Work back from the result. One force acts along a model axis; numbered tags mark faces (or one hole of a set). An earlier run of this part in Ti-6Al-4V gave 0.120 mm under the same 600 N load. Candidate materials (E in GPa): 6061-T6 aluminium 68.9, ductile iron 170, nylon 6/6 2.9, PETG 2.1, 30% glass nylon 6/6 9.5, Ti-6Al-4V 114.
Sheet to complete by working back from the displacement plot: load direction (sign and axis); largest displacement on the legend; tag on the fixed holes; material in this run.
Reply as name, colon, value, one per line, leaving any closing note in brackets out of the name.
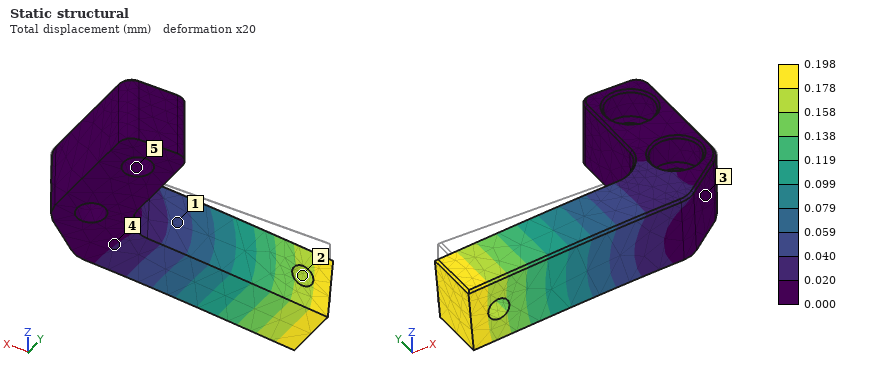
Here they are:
load direction: -Z
largest displacement on the legend: 0.198 mm
tag on the fixed holes: 5
material in this run: 6061-T6 aluminium
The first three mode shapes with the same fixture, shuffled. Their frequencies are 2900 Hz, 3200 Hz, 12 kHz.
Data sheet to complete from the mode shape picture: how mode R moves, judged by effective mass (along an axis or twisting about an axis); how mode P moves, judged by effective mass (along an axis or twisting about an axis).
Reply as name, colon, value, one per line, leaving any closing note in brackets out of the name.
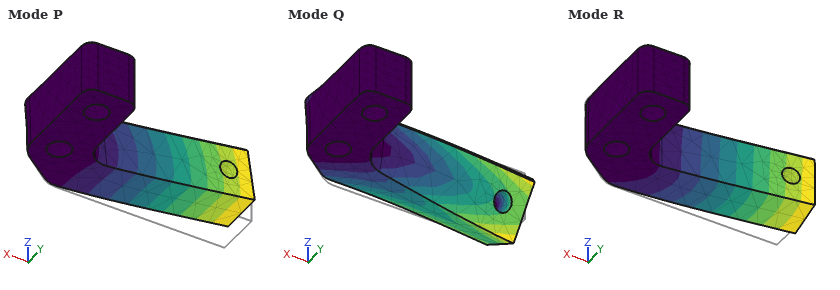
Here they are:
how mode R moves, judged by effective mass: along Y
how mode P moves, judged by effective mass: along Z
